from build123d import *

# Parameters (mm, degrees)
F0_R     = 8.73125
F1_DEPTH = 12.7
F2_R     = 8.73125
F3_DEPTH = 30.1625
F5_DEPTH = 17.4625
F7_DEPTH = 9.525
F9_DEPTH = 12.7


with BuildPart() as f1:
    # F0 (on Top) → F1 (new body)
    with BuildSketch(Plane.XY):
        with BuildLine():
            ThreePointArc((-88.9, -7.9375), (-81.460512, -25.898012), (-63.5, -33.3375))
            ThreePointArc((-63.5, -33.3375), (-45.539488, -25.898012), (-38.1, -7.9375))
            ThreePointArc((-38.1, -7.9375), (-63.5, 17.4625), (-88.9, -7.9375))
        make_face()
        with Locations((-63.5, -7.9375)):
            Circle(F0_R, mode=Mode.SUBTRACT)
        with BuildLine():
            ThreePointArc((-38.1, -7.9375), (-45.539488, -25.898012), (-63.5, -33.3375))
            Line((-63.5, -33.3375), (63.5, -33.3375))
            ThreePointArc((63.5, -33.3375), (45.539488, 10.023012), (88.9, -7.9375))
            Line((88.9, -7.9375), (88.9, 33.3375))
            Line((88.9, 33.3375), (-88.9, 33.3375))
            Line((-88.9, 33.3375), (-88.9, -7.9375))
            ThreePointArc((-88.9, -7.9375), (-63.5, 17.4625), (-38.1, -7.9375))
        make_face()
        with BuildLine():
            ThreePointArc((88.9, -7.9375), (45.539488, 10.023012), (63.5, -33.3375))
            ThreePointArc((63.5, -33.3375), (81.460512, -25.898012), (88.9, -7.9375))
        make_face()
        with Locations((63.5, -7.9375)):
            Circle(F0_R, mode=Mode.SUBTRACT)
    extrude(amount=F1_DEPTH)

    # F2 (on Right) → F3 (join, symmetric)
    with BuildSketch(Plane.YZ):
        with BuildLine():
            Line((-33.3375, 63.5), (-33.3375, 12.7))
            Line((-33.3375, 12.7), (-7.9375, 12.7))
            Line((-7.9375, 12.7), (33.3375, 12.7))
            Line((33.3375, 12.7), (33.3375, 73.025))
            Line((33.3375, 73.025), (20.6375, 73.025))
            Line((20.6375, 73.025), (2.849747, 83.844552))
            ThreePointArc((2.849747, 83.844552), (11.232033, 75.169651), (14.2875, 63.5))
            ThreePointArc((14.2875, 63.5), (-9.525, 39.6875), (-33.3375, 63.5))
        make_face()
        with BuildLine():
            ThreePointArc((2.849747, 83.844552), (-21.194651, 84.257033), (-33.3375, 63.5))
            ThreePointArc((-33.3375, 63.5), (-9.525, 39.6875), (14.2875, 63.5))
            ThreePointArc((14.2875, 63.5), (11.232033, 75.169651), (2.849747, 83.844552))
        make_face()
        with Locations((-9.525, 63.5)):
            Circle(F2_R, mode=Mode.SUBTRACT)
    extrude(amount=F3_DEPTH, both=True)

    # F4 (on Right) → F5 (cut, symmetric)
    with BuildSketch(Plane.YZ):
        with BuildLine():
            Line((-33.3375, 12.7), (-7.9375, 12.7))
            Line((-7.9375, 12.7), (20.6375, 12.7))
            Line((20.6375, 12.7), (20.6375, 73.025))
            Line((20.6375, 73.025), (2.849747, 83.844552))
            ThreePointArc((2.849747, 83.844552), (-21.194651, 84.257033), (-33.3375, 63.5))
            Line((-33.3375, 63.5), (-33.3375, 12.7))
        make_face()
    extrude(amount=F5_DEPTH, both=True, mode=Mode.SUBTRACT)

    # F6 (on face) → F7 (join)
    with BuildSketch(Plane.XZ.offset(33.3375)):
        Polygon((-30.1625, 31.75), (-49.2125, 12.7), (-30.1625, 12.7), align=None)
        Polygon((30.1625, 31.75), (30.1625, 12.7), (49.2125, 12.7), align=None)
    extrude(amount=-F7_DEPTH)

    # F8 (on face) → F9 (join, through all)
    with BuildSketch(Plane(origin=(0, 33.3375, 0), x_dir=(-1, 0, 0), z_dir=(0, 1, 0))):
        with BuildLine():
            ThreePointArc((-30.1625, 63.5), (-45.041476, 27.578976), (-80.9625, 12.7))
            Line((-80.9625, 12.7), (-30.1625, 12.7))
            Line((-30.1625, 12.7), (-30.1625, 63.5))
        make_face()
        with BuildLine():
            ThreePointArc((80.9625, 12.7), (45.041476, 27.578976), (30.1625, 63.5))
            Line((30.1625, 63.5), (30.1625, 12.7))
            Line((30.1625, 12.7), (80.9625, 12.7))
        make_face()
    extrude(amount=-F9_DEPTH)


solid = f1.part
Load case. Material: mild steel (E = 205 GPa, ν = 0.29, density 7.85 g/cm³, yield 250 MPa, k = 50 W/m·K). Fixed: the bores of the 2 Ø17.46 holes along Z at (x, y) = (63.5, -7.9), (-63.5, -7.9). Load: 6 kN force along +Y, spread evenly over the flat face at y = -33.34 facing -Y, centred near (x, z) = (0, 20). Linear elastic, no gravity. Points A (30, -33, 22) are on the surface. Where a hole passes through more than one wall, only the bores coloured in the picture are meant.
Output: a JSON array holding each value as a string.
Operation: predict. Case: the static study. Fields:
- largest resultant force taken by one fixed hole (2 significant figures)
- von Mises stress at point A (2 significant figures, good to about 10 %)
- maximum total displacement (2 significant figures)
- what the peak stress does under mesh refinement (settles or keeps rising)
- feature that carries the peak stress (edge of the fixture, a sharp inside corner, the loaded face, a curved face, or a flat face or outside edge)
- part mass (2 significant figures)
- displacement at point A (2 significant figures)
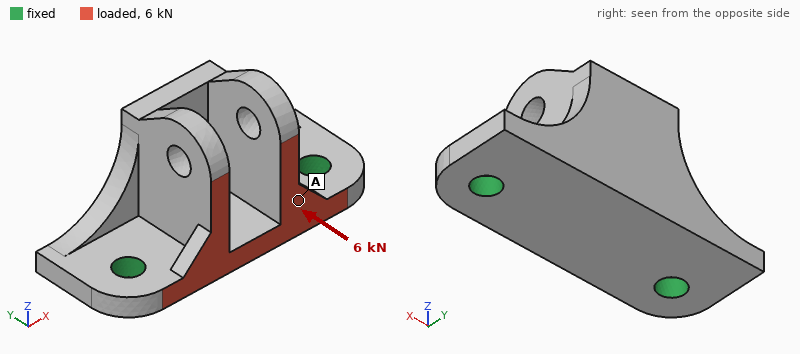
["3.0 kN", "4.2 MPa", "22 µm", "keeps rising", "edge of the fixture", "2.3 kg", "9.4 µm"]
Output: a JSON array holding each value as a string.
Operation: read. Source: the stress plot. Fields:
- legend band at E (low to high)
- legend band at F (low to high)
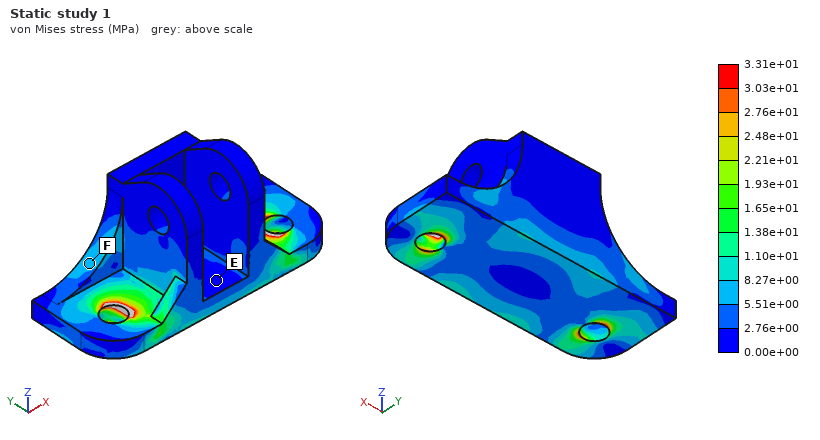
["0.00e+00 to 2.76e+00 MPa", "5.51e+00 to 8.27e+00 MPa"]
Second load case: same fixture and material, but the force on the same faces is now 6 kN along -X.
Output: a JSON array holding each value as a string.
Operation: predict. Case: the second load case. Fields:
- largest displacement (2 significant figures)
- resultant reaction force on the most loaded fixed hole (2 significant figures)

["14 µm", "3.3 kN"]
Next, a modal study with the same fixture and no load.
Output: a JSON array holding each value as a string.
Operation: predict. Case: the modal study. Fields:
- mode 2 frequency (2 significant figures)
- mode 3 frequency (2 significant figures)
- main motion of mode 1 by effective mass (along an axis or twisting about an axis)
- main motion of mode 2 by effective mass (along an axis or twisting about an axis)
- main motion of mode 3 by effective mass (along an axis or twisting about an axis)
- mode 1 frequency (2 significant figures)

["3000 Hz", "3200 Hz", "along Y", "along X", "along Z", "1700 Hz"]
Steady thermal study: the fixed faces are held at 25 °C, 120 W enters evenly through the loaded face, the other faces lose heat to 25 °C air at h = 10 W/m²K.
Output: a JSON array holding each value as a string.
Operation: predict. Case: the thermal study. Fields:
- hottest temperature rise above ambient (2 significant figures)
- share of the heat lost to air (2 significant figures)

["59 K", "13 %"]
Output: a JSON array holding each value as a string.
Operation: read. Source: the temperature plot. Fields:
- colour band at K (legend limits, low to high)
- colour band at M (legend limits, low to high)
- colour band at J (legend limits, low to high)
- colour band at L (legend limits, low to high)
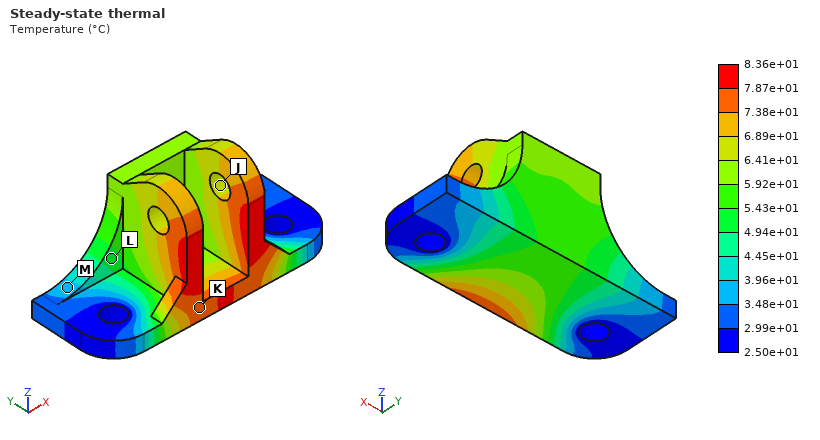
["7.38e+01 to 7.87e+01 °C", "3.48e+01 to 3.96e+01 °C", "6.41e+01 to 6.89e+01 °C", "4.94e+01 to 5.43e+01 °C"]
